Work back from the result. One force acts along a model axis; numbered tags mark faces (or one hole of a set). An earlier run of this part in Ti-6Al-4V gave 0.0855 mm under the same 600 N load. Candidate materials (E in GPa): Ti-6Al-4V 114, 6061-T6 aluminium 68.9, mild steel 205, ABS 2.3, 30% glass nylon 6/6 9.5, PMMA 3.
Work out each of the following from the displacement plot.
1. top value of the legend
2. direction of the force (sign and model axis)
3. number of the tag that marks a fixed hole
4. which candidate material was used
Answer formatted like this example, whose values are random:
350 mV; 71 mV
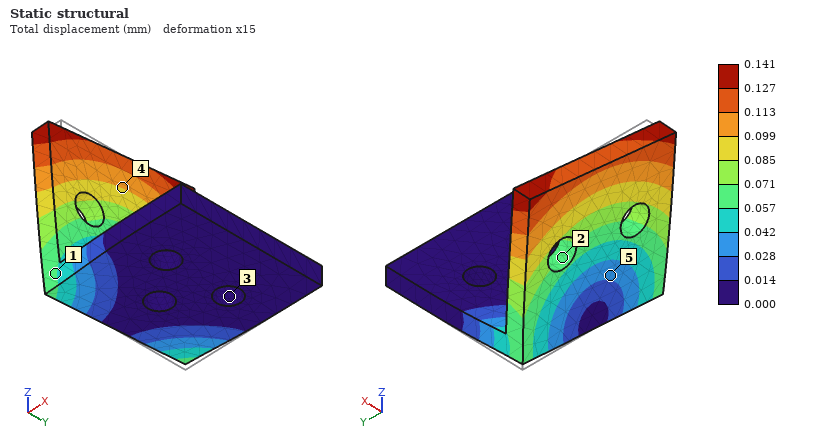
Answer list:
0.141 mm; -Y; 3; 6061-T6 aluminium
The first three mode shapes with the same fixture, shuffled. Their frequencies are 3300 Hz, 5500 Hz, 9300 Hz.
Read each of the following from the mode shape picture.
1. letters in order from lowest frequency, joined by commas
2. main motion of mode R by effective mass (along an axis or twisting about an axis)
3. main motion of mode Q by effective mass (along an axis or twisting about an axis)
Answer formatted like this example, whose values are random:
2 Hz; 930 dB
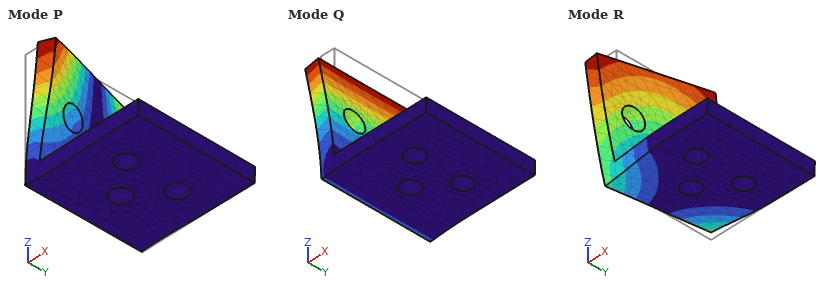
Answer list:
Q, R, P; along Y; along X
